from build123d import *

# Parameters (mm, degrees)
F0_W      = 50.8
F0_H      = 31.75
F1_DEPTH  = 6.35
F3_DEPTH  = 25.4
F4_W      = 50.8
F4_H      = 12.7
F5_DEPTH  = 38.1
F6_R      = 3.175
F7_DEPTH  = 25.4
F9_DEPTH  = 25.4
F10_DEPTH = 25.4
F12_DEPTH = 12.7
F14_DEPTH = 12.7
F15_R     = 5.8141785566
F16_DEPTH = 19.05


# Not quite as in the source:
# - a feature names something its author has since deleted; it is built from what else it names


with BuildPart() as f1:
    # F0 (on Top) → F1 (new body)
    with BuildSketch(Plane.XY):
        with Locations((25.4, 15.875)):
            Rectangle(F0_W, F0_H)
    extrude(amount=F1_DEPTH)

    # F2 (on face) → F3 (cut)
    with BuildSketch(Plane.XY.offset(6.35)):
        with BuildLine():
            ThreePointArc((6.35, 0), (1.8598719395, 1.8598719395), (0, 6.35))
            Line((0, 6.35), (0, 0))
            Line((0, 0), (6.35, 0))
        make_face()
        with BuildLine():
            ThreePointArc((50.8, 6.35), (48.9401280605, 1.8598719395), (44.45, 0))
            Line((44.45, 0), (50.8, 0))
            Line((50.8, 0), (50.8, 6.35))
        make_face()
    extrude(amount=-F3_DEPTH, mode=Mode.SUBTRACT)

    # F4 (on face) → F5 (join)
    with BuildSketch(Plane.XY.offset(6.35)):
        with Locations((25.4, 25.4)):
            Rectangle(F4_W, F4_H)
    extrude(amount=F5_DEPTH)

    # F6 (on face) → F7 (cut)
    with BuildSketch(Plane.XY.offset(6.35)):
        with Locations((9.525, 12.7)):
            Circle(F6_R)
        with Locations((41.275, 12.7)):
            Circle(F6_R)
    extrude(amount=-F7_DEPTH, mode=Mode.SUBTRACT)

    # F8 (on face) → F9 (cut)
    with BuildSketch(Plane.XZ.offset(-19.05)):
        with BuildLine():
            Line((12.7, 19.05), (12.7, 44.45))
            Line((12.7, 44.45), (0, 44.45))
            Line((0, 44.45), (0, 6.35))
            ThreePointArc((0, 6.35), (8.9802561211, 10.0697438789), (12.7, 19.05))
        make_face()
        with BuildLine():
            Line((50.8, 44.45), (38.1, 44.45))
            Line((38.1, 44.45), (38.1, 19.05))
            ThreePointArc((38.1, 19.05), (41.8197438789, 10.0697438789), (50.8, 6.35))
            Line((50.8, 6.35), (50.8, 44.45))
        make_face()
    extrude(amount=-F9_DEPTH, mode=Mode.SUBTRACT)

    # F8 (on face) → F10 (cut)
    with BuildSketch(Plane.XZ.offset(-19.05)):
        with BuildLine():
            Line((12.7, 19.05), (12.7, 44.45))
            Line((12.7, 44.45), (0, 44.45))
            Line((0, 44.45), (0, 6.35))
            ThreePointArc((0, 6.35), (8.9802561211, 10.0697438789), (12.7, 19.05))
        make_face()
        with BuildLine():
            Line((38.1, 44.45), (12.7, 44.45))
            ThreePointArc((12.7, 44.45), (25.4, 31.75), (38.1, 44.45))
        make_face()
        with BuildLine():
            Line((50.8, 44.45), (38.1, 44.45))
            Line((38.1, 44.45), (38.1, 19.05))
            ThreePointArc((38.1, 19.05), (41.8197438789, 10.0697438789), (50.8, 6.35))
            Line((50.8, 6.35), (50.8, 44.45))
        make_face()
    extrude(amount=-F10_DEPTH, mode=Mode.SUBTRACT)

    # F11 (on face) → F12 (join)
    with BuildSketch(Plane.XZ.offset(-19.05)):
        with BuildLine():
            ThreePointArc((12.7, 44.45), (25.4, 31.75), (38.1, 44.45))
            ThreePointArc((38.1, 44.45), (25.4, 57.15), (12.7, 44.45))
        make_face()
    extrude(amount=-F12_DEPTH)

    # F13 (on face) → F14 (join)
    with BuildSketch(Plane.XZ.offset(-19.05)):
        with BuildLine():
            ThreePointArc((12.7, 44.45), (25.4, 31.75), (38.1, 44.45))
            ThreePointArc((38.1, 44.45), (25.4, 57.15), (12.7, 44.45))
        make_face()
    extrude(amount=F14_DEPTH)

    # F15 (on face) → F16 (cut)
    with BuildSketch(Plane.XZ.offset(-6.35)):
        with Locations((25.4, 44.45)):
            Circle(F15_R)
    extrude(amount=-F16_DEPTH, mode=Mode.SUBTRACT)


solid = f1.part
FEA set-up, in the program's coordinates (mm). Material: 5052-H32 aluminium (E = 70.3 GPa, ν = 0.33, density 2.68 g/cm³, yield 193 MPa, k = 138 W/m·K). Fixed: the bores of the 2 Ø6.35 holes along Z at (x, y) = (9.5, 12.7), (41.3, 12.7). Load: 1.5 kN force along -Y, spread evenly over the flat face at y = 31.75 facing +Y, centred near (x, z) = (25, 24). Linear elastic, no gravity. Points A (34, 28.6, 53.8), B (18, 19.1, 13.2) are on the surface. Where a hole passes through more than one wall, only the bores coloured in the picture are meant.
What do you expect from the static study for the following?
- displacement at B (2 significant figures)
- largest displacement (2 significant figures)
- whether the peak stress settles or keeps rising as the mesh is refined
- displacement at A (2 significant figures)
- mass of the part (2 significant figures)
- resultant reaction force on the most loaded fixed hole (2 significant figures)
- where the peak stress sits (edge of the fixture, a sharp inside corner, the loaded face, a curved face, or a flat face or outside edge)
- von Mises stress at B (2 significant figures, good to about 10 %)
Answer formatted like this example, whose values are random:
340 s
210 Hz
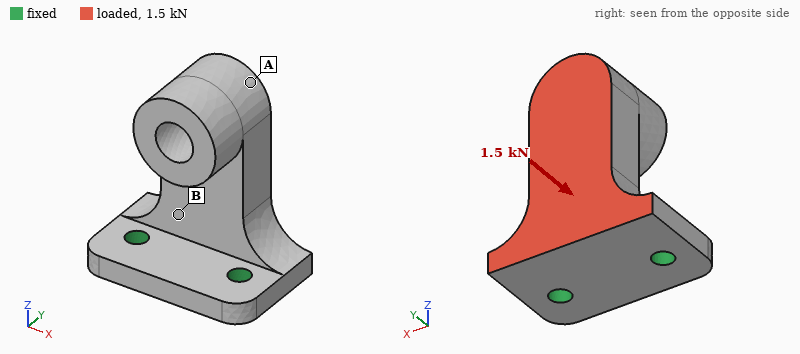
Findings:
0.041 mm
0.27 mm
keeps rising
0.25 mm
82 g
780 N
edge of the fixture
28 MPa
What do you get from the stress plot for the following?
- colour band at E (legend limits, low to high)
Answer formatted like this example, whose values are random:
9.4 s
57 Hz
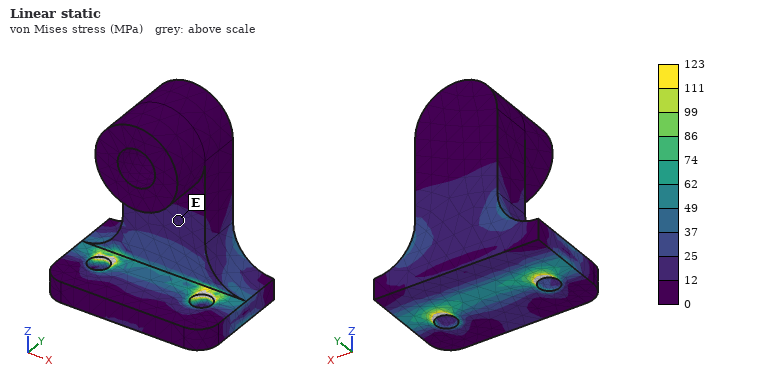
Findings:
12 to 25 MPa
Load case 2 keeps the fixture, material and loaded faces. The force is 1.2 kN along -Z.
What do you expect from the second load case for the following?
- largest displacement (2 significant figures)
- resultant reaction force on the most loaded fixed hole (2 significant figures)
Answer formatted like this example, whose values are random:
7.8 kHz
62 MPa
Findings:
0.13 mm
600 N
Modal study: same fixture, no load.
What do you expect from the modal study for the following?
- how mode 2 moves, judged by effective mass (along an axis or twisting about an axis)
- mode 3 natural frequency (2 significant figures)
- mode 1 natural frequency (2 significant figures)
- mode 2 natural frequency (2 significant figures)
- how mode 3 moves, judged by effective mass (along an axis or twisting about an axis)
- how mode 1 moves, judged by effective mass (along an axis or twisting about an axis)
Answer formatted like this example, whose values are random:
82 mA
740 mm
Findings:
along X
7600 Hz
1600 Hz
3900 Hz
along Z
along Y
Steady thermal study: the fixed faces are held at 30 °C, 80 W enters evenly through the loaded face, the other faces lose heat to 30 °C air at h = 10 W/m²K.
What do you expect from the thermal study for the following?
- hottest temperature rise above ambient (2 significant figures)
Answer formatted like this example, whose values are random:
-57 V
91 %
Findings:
54 K
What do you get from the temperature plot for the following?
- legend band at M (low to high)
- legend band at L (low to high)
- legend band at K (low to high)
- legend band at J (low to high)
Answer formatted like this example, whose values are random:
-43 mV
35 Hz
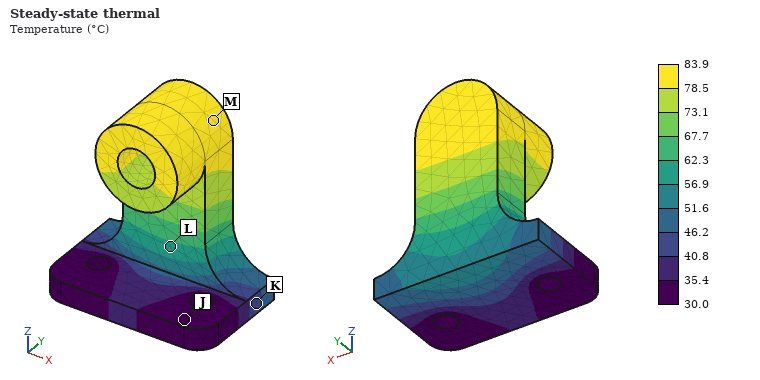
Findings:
78.5 to 83.9 °C
56.9 to 62.3 °C
40.8 to 46.2 °C
30.0 to 35.4 °C
